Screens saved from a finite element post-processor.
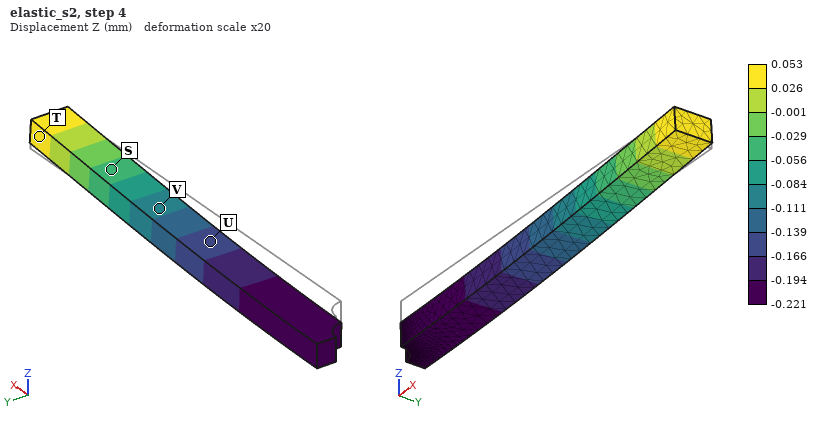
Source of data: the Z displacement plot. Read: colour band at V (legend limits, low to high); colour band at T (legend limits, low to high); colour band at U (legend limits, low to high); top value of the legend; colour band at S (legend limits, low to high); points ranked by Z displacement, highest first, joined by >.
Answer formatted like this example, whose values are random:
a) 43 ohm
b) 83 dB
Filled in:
a) -0.111 to -0.084 mm
b) 0.026 to 0.053 mm
c) -0.166 to -0.139 mm
d) 0.053 mm
e) -0.056 to -0.029 mm
f) T > S > V > U
